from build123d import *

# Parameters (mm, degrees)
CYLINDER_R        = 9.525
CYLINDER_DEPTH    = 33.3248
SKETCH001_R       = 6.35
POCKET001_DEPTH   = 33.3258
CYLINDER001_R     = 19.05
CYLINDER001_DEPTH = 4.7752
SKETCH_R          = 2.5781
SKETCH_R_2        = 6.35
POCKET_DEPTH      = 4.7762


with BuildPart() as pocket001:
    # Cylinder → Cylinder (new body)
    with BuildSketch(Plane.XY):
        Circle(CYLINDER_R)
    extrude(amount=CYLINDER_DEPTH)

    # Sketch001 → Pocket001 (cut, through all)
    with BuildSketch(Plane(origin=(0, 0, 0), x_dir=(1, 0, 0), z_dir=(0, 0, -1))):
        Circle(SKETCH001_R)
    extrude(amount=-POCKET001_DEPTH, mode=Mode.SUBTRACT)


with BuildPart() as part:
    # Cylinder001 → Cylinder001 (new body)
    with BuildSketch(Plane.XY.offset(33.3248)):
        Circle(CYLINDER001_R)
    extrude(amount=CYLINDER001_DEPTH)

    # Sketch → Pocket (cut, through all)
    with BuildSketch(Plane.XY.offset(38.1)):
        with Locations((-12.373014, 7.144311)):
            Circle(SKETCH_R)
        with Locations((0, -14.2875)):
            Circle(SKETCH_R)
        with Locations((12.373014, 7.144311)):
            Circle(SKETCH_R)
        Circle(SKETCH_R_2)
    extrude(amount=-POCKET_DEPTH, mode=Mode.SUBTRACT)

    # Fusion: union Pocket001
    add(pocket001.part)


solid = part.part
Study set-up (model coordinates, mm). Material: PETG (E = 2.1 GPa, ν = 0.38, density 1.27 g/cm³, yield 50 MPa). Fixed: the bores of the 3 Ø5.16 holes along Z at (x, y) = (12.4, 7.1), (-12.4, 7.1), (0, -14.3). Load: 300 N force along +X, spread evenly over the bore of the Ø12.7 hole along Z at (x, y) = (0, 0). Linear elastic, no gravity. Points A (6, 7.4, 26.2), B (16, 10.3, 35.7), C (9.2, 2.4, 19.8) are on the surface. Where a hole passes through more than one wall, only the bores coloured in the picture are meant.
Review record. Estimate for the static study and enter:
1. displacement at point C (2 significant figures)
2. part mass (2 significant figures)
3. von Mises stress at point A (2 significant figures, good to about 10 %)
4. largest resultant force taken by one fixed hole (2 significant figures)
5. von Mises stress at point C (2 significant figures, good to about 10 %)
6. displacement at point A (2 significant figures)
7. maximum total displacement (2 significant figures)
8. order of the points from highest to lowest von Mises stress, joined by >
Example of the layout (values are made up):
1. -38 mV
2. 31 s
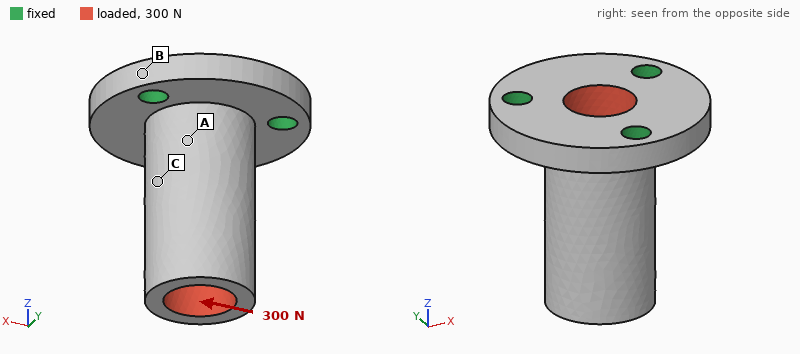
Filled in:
1. 0.17 mm
2. 12 g
3. 4.4 MPa
4. 240 N
5. 2.7 MPa
6. 0.085 mm
7. 0.36 mm
8. A > C > B
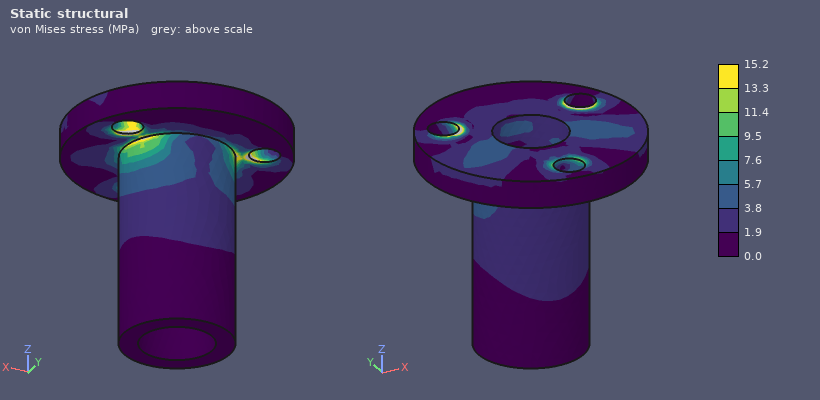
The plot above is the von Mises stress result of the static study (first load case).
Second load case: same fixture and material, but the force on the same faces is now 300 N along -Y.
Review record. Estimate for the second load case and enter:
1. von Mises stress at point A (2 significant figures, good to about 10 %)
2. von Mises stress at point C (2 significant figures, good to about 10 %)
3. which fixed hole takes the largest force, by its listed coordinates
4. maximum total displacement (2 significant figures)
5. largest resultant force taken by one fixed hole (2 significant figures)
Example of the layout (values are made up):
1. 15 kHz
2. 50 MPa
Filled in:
1. 3.5 MPa
2. 2.9 MPa
3. (0, -14.3)
4. 0.36 mm
5. 270 N
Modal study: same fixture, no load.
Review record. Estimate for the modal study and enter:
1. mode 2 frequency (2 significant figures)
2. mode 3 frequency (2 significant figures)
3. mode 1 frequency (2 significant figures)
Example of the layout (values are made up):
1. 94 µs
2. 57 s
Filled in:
1. 2000 Hz
2. 5400 Hz
3. 2000 Hz
